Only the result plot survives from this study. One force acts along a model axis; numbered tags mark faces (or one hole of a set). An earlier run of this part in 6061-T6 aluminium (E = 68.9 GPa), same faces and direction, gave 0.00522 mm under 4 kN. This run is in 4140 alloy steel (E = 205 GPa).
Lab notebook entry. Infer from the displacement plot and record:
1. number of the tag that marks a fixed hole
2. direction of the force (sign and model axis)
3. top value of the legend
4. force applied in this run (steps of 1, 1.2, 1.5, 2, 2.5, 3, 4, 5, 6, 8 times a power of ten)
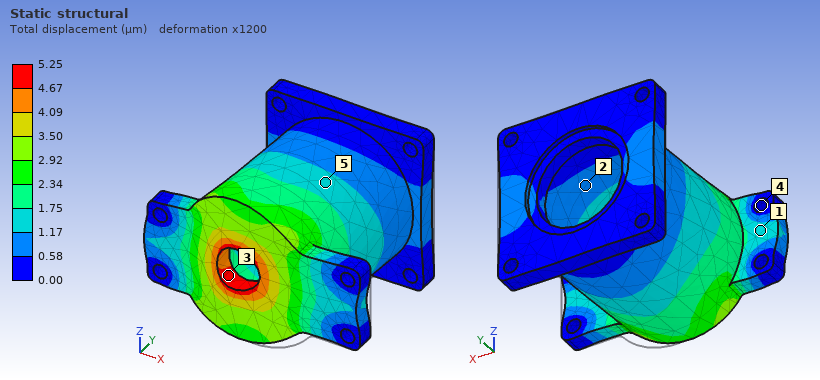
4
-X
5.25 µm
12 kN
